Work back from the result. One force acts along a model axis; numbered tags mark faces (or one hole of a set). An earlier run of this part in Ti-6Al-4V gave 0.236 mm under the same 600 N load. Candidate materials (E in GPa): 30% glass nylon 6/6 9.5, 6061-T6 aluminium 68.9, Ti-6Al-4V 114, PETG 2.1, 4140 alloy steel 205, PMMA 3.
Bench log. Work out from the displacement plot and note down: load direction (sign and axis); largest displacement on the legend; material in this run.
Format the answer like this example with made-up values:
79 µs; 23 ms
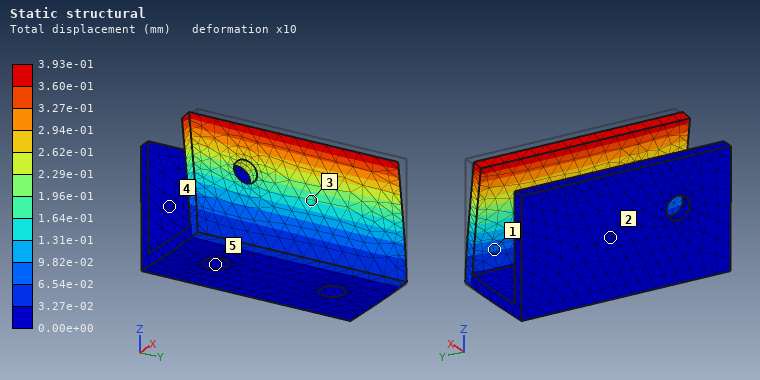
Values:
-X; 3.93e-01 mm; 6061-T6 aluminium
